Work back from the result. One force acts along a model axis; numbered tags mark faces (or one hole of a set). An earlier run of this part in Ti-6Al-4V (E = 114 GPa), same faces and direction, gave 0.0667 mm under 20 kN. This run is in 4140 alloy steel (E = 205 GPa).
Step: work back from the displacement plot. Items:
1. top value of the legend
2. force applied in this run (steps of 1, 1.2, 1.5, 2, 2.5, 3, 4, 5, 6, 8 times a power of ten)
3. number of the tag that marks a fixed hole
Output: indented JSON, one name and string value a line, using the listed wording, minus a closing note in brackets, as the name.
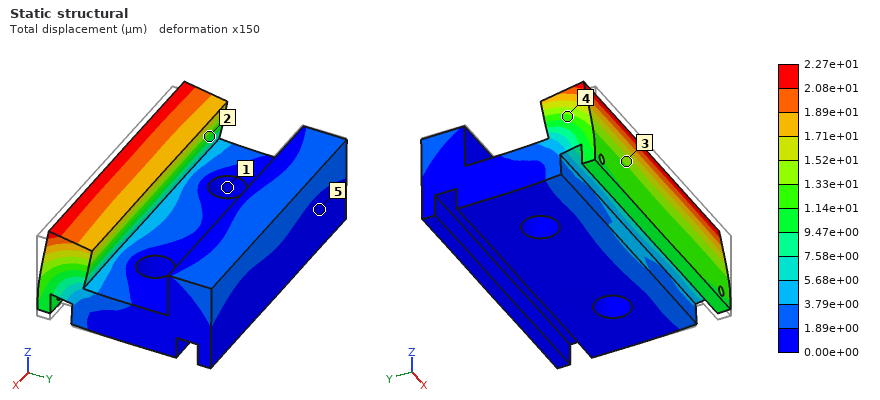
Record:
{
  "top value of the legend": "2.27e+01 µm",
  "force applied in this run": "12 kN",
  "number of the tag that marks a fixed hole": "1"
}
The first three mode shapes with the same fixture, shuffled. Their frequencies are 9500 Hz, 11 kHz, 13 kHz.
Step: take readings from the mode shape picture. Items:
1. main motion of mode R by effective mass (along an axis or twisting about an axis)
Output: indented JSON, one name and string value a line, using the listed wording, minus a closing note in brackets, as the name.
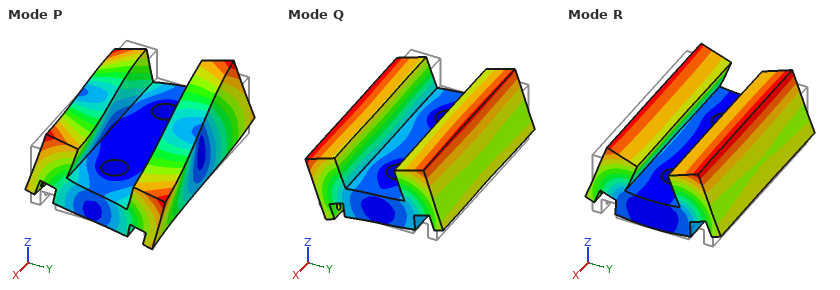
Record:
{
  "main motion of mode R by effective mass": "along Z"
}
